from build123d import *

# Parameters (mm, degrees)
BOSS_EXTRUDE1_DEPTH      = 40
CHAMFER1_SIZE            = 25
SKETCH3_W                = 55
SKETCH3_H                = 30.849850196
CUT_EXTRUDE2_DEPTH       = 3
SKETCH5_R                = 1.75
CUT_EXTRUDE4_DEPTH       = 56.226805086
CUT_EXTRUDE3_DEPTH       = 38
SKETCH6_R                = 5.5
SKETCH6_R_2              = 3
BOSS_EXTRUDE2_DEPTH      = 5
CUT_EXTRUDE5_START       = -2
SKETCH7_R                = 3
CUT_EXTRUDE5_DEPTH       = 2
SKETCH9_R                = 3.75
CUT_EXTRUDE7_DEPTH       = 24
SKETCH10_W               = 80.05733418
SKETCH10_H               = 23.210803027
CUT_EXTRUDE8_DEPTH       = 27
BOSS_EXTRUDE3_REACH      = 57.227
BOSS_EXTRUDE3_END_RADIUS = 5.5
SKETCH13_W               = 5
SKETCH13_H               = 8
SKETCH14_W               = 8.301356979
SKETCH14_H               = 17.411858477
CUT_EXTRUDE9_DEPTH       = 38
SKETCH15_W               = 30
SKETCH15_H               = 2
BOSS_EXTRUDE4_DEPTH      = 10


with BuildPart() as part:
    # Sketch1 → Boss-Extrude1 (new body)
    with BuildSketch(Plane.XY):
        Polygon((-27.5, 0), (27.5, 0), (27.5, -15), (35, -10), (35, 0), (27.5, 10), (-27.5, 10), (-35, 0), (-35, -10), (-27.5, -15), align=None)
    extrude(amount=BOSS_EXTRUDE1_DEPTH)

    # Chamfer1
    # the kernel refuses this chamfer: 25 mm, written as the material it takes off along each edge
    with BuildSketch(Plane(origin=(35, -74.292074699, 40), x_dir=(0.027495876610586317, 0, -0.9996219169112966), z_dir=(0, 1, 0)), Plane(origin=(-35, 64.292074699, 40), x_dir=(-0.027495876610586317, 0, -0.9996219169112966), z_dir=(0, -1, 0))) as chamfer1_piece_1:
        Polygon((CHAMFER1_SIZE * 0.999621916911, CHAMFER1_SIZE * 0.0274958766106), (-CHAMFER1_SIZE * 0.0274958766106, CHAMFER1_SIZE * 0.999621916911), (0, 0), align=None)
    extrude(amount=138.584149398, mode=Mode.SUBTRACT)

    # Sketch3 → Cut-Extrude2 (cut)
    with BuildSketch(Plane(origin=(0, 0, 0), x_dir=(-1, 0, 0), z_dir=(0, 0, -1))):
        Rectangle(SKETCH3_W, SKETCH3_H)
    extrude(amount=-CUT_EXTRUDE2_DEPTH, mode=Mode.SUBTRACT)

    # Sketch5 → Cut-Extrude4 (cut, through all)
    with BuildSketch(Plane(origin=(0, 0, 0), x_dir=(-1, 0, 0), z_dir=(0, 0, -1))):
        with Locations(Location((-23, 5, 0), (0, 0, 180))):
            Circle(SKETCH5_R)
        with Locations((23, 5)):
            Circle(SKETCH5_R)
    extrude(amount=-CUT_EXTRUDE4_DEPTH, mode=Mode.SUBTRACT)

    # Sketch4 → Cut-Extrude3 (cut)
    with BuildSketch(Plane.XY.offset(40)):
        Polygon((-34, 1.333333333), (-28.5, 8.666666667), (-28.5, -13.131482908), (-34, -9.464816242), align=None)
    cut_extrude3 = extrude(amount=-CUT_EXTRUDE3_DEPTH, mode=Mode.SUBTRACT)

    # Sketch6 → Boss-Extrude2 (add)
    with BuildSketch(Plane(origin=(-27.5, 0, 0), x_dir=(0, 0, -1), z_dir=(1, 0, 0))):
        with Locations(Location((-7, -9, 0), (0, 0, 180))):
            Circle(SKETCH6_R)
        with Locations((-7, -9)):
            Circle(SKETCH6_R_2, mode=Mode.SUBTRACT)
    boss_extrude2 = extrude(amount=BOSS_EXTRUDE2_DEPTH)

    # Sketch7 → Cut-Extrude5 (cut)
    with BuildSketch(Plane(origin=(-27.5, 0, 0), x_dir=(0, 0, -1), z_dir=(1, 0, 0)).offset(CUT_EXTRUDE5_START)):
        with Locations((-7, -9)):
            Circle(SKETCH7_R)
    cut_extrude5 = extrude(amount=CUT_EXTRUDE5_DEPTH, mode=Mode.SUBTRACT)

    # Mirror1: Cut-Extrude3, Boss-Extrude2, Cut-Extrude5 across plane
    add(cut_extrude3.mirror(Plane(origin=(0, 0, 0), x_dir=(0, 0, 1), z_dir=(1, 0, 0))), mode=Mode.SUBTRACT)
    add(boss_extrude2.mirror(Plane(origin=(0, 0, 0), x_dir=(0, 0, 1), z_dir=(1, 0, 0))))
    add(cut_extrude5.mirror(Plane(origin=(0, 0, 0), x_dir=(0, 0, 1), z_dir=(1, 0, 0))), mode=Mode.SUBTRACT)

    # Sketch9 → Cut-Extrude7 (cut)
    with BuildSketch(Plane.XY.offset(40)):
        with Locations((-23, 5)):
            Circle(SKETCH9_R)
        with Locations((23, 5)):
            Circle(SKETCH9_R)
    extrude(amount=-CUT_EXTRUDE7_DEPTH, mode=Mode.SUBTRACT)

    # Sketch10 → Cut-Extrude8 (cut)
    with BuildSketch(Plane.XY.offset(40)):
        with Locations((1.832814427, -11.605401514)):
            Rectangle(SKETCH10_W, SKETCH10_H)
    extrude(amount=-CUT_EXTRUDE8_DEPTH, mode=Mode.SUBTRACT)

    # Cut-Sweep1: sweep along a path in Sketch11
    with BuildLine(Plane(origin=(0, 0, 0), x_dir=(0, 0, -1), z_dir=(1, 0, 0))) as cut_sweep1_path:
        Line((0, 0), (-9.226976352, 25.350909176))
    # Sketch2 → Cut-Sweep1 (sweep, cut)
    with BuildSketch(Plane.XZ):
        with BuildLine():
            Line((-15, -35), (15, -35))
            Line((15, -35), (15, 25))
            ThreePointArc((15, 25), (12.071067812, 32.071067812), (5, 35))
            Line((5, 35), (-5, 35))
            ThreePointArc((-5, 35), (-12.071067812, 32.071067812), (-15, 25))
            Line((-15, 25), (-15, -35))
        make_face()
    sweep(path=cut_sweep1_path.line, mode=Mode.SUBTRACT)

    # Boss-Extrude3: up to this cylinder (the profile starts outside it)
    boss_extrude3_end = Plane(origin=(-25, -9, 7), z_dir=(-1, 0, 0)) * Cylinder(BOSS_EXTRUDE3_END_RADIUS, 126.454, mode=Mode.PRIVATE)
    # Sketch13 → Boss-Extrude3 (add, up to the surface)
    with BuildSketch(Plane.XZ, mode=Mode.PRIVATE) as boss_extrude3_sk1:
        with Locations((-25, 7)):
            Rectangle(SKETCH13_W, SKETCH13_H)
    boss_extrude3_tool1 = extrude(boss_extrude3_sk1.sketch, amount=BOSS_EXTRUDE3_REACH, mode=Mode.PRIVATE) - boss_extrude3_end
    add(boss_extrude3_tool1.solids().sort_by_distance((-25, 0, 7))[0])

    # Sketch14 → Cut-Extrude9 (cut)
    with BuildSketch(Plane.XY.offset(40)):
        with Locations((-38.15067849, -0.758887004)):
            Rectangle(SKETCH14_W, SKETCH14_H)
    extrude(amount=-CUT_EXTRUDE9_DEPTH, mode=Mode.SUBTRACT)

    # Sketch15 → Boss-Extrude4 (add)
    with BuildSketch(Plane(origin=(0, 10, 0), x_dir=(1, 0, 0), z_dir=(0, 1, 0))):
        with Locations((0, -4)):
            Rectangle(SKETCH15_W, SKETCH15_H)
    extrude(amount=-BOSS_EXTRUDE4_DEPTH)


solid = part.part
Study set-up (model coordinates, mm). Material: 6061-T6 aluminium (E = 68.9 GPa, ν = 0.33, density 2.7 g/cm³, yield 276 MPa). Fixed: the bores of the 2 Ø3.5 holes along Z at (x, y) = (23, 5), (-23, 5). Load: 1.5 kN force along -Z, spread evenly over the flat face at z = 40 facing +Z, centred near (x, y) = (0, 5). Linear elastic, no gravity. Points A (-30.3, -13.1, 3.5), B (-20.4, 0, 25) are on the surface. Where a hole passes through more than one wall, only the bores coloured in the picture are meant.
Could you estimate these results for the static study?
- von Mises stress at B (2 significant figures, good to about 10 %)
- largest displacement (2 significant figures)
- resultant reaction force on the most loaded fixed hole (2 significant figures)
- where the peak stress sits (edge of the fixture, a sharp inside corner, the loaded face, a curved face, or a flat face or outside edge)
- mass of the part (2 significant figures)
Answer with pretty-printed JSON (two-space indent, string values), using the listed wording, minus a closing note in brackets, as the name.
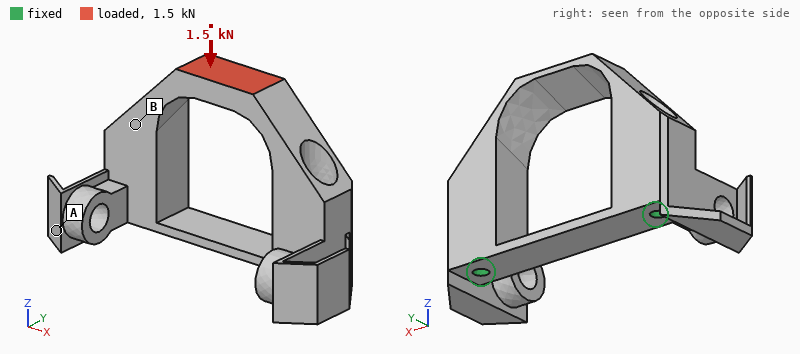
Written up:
{
  "von Mises stress at B": "31 MPa",
  "largest displacement": "90 µm",
  "resultant reaction force on the most loaded fixed hole": "980 N",
  "where the peak stress sits": "the loaded face",
  "mass of the part": "25 g"
}
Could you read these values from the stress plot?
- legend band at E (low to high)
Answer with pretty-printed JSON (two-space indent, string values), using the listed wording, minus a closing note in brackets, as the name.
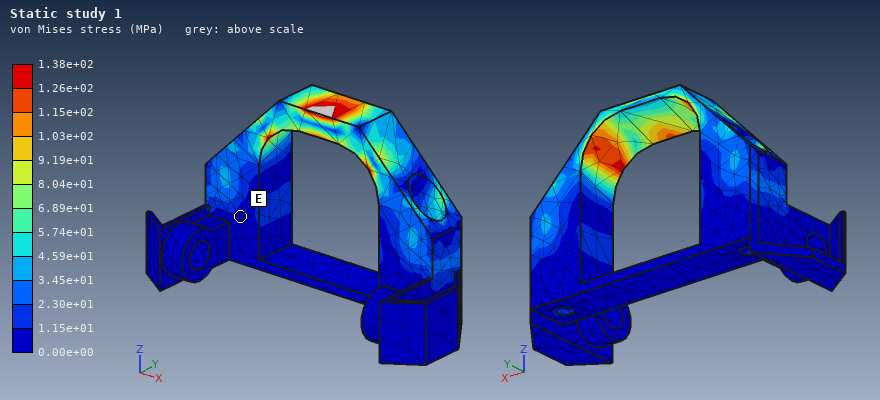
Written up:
{
  "legend band at E": "0.00e+00 to 1.15e+01 MPa"
}
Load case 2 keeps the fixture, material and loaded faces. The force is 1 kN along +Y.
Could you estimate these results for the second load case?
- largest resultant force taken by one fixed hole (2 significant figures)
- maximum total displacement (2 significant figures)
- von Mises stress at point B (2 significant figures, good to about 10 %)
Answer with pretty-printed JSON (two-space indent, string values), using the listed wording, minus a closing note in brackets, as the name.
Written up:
{
  "largest resultant force taken by one fixed hole": "500 N",
  "maximum total displacement": "0.17 mm",
  "von Mises stress at point B": "64 MPa"
}
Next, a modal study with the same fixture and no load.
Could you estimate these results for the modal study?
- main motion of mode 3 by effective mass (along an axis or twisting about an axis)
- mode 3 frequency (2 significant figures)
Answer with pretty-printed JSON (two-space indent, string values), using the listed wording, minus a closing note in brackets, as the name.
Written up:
{
  "main motion of mode 3 by effective mass": "along Y",
  "mode 3 frequency": "8200 Hz"
}
